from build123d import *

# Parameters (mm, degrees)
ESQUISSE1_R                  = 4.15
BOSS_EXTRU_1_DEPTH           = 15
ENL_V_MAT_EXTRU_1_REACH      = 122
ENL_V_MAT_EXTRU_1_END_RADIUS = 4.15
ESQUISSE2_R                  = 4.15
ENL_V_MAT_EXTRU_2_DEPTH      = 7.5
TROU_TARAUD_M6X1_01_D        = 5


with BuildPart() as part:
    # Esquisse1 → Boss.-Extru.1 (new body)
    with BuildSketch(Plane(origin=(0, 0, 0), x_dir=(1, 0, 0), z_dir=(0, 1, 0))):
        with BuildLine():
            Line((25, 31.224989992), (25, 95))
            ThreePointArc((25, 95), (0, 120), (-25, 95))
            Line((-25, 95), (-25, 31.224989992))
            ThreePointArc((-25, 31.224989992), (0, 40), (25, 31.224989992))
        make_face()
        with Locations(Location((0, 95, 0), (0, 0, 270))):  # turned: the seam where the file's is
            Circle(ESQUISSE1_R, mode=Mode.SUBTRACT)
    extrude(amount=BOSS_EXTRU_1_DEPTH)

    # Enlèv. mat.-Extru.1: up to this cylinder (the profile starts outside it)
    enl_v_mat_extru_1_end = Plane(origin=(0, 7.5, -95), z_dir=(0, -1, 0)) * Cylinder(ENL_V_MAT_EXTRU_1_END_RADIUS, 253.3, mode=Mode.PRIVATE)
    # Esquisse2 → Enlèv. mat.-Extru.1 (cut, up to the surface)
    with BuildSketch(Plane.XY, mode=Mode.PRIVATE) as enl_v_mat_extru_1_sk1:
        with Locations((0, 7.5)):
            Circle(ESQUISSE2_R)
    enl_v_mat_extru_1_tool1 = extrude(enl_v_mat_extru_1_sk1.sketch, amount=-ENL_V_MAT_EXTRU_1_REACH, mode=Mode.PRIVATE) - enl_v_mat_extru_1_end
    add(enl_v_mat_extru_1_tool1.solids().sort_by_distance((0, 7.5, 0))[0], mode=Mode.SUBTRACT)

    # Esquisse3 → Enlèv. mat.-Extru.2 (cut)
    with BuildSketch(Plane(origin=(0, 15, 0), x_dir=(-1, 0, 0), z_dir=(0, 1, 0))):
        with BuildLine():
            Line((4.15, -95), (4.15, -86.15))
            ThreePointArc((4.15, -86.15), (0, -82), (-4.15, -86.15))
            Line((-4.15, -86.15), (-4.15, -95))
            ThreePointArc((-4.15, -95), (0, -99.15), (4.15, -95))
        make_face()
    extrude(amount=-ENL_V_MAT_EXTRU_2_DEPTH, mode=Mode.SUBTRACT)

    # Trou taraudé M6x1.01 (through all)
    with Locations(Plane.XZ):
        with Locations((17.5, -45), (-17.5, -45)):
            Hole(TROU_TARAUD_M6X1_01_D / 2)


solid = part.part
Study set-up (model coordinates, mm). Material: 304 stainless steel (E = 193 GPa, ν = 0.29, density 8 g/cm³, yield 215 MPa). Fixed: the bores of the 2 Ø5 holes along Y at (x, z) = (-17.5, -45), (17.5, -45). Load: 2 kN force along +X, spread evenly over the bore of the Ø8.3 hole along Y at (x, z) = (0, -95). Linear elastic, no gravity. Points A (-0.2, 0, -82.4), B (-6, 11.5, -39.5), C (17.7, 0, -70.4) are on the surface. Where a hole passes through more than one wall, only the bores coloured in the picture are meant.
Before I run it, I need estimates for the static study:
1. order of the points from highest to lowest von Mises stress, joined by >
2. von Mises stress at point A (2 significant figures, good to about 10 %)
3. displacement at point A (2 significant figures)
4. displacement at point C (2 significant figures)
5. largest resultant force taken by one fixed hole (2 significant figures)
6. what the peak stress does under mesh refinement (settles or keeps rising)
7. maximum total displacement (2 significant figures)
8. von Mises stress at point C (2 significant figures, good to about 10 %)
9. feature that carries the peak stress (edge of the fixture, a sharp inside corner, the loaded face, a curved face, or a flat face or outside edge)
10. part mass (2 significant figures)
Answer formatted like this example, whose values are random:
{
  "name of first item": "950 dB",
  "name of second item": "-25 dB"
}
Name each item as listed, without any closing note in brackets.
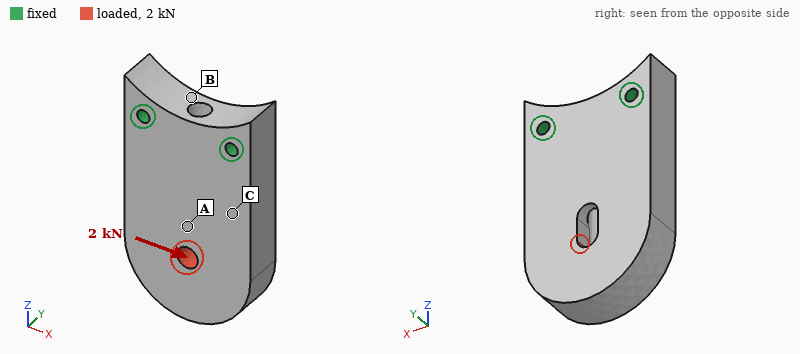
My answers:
{
  "order of the points from highest to lowest von Mises stress, joined by >": "A > C > B",
  "von Mises stress at point A": "17 MPa",
  "displacement at point A": "4.2 µm",
  "displacement at point C": "2.8 µm",
  "largest resultant force taken by one fixed hole": "2.9 kN",
  "what the peak stress does under mesh refinement": "keeps rising",
  "maximum total displacement": "8.7 µm",
  "von Mises stress at point C": "7.6 MPa",
  "feature that carries the peak stress": "edge of the fixture",
  "part mass": "430 g"
}
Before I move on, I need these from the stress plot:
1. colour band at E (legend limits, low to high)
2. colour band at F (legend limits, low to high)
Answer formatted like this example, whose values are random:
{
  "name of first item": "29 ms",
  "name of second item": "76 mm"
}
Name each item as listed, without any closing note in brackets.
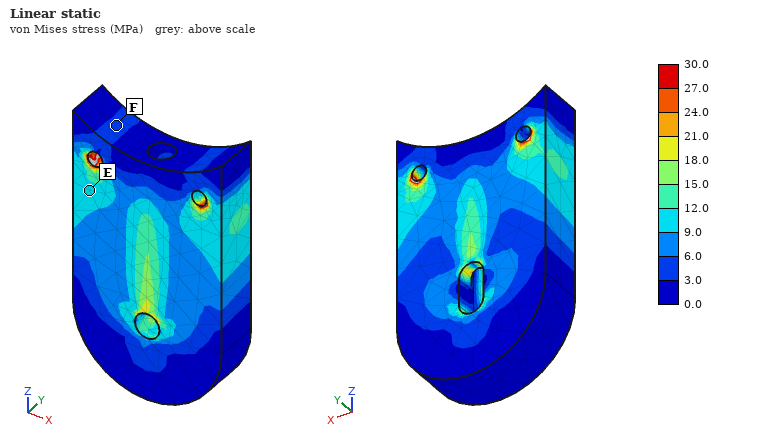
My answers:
{
  "colour band at E": "9.0 to 12.0 MPa",
  "colour band at F": "3.0 to 6.0 MPa"
}
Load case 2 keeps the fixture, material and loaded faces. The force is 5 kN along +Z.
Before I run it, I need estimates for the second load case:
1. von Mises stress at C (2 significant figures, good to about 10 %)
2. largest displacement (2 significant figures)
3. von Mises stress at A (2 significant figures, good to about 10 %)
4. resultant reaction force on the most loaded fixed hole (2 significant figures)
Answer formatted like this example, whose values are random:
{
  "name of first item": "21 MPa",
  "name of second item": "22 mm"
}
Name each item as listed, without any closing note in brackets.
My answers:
{
  "von Mises stress at C": "10 MPa",
  "largest displacement": "6.7 µm",
  "von Mises stress at A": "16 MPa",
  "resultant reaction force on the most loaded fixed hole": "2.5 kN"
}
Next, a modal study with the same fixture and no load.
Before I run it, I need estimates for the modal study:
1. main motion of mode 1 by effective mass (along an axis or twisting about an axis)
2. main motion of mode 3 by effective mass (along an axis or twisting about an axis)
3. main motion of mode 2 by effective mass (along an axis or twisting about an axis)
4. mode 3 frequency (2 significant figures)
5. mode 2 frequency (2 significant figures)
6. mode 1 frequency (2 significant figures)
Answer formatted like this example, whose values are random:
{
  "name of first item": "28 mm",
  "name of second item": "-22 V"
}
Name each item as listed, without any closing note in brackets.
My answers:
{
  "main motion of mode 1 by effective mass": "along Y",
  "main motion of mode 3 by effective mass": "twisting about Z",
  "main motion of mode 2 by effective mass": "along X",
  "mode 3 frequency": "6800 Hz",
  "mode 2 frequency": "5800 Hz",
  "mode 1 frequency": "2200 Hz"
}
